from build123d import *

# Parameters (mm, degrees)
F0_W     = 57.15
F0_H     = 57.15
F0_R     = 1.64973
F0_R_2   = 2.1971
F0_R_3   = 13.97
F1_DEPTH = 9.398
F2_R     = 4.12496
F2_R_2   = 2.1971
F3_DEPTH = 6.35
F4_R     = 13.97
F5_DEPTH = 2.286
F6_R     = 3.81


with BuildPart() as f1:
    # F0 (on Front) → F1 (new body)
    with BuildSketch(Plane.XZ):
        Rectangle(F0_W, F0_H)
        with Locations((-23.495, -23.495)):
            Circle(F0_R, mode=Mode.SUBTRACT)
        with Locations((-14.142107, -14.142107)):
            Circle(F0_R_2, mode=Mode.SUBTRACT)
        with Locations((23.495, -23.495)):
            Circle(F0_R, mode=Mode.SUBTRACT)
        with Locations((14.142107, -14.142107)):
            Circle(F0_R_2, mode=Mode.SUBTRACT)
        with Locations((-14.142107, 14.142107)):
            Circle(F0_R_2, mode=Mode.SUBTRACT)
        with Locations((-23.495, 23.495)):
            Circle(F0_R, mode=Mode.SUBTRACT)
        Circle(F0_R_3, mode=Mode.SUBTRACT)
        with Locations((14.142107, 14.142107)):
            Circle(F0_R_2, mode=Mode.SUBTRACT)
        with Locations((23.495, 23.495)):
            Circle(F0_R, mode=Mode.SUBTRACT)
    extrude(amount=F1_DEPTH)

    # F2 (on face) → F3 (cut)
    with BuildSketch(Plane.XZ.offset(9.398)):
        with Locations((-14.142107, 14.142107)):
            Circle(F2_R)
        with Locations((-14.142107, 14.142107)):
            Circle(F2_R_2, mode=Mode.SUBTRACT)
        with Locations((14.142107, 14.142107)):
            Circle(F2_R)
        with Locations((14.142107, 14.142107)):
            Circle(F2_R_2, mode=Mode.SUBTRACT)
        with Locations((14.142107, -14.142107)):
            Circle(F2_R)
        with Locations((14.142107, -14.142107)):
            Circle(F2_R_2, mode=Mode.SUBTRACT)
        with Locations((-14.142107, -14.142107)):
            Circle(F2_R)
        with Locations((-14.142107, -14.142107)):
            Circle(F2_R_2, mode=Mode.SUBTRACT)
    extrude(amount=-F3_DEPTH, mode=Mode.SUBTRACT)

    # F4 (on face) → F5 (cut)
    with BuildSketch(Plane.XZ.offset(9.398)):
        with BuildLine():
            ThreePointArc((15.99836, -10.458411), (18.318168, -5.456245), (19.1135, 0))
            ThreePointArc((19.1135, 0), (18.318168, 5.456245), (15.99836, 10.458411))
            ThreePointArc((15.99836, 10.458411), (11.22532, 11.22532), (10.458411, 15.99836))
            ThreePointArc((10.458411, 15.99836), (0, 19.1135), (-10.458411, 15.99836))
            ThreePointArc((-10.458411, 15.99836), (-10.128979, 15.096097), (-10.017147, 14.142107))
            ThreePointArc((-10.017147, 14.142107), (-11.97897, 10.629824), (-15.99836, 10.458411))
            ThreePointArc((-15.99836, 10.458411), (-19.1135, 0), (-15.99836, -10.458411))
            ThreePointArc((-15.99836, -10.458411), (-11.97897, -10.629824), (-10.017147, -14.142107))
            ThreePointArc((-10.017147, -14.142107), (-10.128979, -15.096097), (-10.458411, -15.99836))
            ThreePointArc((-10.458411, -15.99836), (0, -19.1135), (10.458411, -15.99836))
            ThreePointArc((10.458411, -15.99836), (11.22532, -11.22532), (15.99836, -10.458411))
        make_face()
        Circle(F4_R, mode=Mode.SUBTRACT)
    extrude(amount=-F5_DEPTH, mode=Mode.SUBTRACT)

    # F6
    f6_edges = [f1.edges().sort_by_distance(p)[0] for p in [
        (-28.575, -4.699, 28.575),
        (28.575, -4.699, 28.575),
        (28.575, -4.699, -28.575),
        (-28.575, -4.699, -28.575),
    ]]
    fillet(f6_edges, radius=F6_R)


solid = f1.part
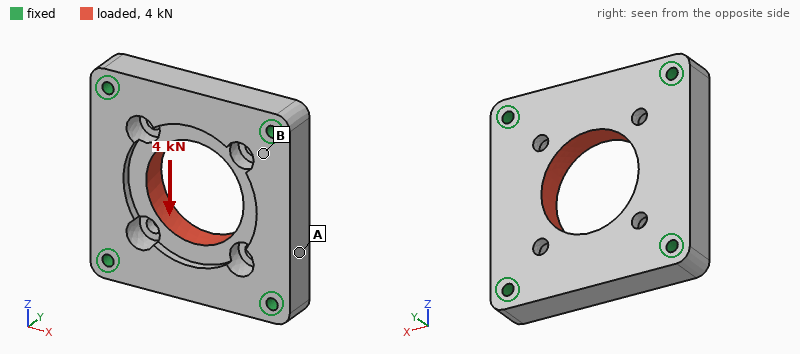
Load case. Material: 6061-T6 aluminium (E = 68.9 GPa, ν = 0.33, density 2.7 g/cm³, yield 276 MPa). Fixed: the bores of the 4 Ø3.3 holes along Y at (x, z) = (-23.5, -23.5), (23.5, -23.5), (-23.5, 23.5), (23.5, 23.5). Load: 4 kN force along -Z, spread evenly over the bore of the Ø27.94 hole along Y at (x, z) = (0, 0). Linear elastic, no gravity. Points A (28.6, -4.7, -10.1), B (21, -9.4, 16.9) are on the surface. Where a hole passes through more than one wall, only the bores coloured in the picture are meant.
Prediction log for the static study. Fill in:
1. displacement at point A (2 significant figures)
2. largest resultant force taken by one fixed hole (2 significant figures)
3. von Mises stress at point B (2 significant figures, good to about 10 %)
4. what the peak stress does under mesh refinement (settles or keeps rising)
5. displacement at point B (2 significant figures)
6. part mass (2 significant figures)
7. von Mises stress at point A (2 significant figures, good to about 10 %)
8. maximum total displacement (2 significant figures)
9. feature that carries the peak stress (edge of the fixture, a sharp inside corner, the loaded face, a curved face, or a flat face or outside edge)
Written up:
1.2 µm
1.1 kN
12 MPa
keeps rising
1.2 µm
59 g
4.0 MPa
6.4 µm
edge of the fixture
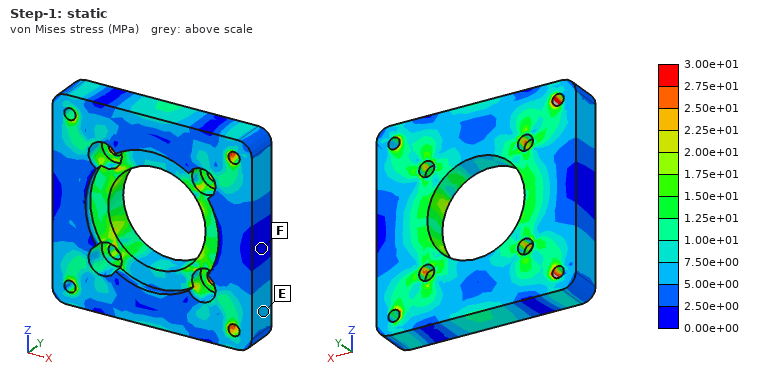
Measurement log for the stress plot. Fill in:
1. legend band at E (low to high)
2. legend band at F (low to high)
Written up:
5.00e+00 to 7.50e+00 MPa
0.00e+00 to 2.50e+00 MPa
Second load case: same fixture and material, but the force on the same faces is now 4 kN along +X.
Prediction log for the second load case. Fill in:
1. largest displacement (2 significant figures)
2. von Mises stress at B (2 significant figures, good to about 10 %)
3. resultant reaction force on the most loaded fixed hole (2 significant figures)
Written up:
6.4 µm
7.0 MPa
1.1 kN
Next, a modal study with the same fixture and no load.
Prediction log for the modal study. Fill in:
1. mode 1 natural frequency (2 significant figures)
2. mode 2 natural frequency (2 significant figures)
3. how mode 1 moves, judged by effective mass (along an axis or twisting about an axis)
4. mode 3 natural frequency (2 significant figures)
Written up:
14 kHz
17 kHz
along Y
17 kHz
